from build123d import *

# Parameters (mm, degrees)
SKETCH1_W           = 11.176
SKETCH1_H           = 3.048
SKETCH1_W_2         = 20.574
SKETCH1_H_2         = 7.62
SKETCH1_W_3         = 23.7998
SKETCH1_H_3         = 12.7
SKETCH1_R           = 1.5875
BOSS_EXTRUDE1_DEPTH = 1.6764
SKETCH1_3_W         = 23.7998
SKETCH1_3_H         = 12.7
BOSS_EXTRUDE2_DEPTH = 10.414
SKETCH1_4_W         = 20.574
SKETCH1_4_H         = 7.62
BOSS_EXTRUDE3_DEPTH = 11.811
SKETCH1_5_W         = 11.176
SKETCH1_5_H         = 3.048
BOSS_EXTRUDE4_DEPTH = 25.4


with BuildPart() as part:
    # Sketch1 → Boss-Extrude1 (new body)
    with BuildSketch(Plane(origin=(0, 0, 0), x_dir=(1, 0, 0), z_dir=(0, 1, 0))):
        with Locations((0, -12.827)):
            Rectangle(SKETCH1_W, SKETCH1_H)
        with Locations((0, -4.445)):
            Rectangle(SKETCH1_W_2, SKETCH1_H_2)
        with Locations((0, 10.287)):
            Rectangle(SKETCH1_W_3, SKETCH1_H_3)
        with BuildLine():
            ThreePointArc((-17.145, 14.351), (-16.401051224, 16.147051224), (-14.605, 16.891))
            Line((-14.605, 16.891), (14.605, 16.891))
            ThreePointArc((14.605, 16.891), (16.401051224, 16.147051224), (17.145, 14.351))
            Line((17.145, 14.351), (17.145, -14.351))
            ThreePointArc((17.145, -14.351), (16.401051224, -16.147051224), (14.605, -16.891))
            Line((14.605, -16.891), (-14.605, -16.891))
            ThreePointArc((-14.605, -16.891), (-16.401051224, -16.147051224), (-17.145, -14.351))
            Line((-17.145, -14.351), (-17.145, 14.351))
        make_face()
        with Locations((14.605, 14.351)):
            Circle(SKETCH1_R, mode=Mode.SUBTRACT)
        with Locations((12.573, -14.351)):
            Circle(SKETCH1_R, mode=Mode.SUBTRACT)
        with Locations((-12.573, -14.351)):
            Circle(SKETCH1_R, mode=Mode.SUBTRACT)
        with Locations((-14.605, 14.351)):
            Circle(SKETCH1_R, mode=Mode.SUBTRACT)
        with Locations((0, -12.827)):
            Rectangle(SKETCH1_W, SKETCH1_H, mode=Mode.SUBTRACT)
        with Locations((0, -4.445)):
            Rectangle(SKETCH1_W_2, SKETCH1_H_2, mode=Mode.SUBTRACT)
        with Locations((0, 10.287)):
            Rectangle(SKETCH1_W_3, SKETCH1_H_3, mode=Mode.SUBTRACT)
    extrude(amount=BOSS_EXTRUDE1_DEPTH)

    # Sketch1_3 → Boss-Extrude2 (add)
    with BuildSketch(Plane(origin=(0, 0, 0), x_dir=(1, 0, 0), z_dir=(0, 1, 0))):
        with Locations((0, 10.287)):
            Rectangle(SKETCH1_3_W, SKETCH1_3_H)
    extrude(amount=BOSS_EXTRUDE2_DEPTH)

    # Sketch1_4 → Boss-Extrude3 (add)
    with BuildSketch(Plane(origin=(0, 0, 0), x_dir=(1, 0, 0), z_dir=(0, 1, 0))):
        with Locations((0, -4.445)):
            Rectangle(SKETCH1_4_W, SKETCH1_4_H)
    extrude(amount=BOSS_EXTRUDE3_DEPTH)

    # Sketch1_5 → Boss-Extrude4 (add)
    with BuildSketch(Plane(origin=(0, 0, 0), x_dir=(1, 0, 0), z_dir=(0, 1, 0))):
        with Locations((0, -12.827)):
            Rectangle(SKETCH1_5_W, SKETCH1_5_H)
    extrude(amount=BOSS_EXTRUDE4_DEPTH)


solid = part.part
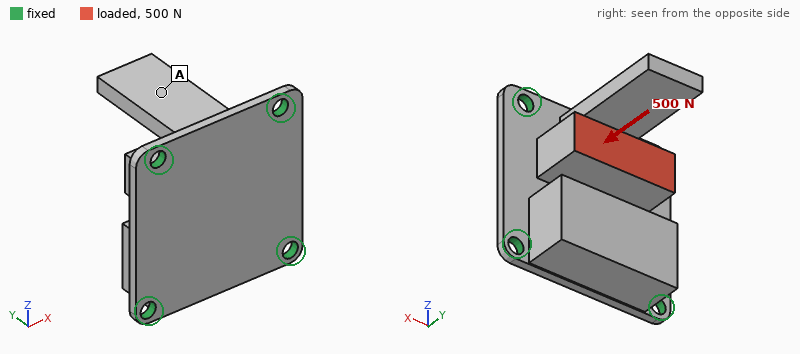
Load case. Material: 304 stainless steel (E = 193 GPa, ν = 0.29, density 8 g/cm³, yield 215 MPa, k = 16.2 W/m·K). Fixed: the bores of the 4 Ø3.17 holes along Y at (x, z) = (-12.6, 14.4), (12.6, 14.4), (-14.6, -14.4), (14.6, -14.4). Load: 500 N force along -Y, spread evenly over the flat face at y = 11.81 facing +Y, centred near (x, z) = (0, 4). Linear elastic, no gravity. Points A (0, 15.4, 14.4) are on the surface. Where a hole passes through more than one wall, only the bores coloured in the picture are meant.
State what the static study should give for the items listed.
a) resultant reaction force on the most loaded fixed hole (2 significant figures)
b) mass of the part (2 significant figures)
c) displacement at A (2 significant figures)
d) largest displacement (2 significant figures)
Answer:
170 N
55 g
17 µm
30 µm
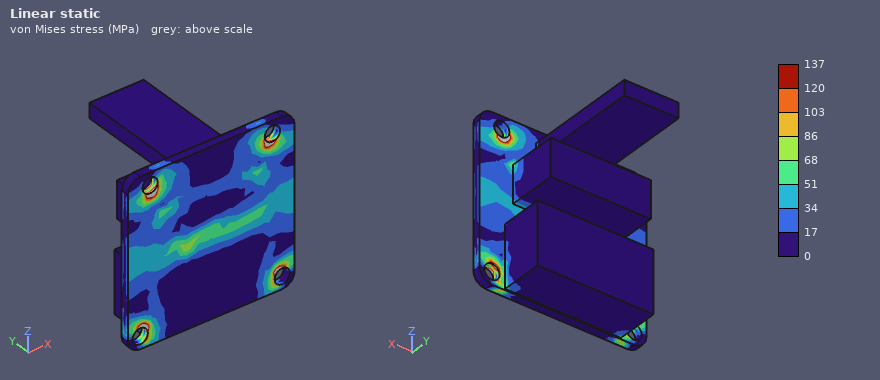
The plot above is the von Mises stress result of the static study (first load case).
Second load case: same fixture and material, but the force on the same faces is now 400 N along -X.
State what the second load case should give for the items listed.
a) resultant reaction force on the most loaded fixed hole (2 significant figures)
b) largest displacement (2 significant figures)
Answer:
160 N
7.7 µm
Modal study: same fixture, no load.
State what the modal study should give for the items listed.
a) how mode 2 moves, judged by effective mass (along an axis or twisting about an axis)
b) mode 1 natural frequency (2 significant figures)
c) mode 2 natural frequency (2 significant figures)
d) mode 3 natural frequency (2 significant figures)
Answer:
along Y
2700 Hz
5300 Hz
6800 Hz
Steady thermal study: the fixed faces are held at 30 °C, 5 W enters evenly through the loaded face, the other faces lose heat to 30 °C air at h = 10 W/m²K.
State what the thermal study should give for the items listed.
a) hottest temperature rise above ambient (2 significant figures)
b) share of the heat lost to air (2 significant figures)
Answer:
54 K
17 %
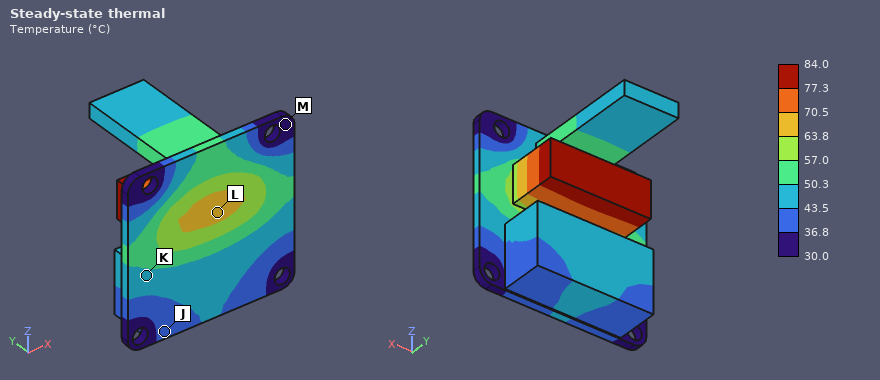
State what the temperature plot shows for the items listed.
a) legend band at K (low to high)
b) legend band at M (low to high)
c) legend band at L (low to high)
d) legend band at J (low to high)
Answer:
43.5 to 50.3 °C
30.0 to 36.8 °C
63.8 to 70.5 °C
36.8 to 43.5 °C
